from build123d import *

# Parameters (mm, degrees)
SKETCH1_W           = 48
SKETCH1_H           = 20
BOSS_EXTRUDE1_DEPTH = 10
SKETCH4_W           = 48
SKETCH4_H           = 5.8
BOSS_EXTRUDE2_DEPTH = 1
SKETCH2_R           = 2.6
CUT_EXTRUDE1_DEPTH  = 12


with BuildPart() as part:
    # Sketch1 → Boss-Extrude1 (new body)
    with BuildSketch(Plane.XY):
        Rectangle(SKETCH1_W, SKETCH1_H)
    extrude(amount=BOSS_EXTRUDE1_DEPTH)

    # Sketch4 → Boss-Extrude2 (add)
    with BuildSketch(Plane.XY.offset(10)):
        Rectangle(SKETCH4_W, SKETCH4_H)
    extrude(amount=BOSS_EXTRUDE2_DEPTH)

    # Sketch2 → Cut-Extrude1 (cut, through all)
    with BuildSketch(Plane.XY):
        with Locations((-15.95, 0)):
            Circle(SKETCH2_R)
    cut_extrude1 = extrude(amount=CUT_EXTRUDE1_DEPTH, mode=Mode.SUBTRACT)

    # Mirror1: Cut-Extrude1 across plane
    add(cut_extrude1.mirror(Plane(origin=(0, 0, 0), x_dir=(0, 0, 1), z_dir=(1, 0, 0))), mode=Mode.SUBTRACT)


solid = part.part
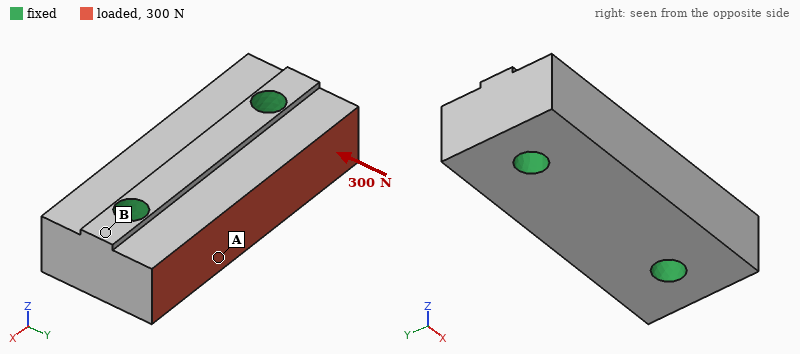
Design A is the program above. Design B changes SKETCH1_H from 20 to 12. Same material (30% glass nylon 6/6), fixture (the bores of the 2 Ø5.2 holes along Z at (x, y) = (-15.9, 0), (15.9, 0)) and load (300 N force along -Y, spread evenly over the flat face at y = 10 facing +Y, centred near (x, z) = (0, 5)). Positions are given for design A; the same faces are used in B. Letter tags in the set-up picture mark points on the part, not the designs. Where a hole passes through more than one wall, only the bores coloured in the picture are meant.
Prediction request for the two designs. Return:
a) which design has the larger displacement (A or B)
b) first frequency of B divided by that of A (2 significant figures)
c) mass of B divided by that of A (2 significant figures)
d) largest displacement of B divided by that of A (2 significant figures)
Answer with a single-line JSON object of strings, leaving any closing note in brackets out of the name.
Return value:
{"which design has the larger displacement": "B", "first frequency of B divided by that of A": "1.1", "mass of B divided by that of A": "0.59", "largest displacement of B divided by that of A": "1.7"}
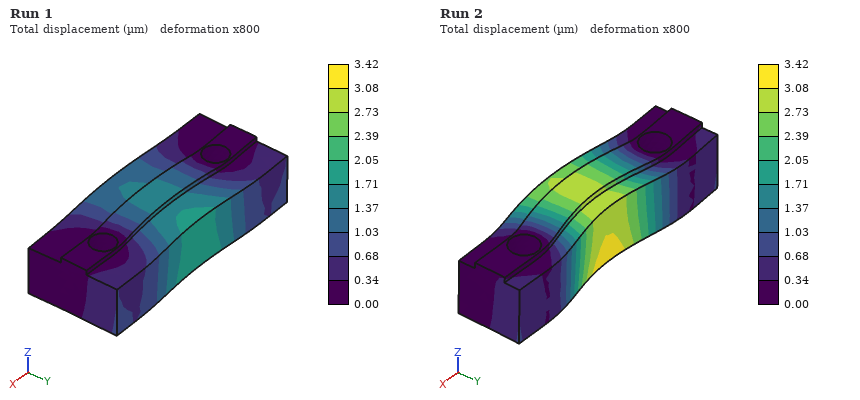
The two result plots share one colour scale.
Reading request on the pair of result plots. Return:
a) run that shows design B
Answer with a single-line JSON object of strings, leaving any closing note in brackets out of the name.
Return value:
{"run that shows design B": "Run 2"}
